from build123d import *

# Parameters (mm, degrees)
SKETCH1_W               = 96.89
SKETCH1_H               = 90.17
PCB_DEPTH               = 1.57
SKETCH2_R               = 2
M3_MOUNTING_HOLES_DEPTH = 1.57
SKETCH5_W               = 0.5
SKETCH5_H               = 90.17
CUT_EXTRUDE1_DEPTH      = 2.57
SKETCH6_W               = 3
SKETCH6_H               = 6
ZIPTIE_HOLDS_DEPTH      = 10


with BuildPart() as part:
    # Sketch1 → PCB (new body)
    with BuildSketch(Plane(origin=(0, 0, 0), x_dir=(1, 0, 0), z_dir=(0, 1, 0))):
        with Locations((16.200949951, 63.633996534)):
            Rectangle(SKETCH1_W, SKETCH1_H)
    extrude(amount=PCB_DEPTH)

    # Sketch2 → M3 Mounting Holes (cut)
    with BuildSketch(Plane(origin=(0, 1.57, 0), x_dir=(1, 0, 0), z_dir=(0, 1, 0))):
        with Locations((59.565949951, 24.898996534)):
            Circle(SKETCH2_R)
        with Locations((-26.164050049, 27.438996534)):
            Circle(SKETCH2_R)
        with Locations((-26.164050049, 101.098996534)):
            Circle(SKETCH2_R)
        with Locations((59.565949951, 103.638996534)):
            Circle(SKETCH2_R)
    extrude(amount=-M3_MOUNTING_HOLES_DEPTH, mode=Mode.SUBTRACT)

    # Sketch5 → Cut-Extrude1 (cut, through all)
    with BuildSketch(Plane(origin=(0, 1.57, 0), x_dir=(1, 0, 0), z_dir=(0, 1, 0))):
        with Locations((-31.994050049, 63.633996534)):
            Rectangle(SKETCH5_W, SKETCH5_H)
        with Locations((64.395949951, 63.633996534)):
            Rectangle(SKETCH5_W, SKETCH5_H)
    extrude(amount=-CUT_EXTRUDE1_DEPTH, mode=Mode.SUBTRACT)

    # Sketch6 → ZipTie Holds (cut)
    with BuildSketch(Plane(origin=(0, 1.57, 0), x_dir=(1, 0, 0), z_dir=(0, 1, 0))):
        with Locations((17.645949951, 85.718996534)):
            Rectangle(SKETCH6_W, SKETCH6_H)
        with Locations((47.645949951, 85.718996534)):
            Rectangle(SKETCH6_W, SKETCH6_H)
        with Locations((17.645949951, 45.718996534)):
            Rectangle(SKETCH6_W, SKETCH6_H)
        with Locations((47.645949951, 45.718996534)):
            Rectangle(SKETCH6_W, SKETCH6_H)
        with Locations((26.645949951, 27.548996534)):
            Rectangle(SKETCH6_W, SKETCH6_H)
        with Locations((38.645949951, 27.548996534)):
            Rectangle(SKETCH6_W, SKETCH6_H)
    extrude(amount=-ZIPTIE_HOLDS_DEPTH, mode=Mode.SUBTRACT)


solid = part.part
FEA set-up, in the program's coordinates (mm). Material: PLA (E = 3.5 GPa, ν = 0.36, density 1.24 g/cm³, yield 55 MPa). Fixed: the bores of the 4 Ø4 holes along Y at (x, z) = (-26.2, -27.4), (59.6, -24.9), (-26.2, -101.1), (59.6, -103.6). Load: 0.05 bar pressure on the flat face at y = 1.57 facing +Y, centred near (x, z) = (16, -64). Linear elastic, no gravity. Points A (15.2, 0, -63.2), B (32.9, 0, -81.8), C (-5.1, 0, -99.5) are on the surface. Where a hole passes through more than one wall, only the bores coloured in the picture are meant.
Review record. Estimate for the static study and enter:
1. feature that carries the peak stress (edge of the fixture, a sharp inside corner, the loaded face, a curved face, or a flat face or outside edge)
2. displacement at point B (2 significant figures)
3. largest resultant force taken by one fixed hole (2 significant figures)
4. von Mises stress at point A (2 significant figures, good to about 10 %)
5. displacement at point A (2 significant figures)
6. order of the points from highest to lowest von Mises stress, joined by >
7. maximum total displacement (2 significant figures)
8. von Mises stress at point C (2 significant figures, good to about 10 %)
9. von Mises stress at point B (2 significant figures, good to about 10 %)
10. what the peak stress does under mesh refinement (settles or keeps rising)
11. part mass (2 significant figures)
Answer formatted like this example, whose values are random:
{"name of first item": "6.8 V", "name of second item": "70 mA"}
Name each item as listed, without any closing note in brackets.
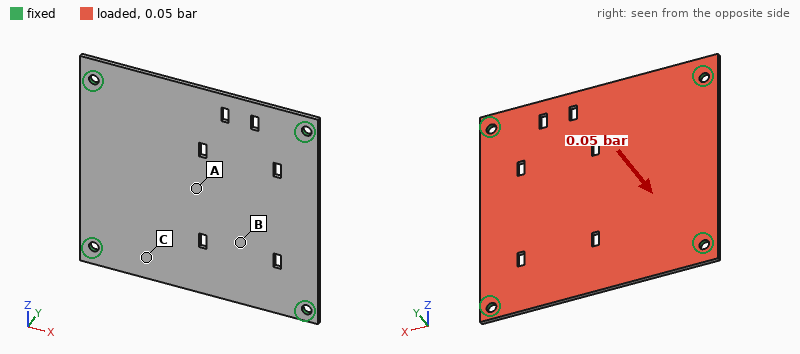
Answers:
{"feature that carries the peak stress": "edge of the fixture", "displacement at point B": "1.0 mm", "largest resultant force taken by one fixed hole": "11 N", "von Mises stress at point A": "4.6 MPa", "displacement at point A": "1.3 mm", "order of the points from highest to lowest von Mises stress, joined by >": "A > B > C", "maximum total displacement": "1.3 mm", "von Mises stress at point C": "1.6 MPa", "von Mises stress at point B": "3.4 MPa", "what the peak stress does under mesh refinement": "keeps rising", "part mass": "17 g"}
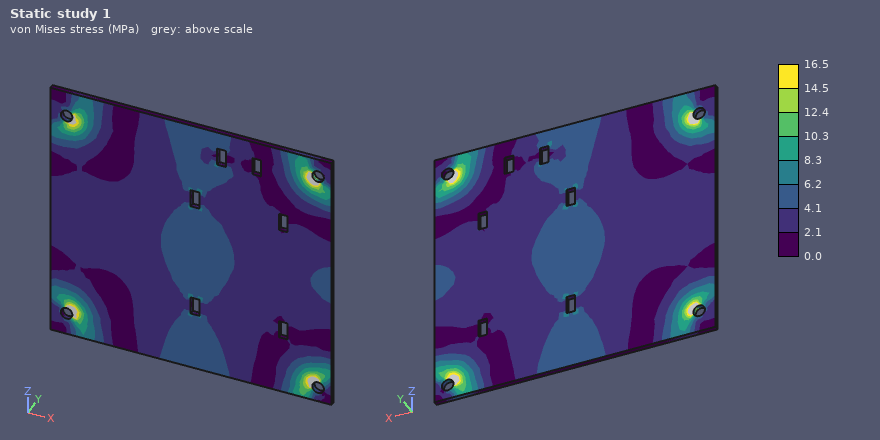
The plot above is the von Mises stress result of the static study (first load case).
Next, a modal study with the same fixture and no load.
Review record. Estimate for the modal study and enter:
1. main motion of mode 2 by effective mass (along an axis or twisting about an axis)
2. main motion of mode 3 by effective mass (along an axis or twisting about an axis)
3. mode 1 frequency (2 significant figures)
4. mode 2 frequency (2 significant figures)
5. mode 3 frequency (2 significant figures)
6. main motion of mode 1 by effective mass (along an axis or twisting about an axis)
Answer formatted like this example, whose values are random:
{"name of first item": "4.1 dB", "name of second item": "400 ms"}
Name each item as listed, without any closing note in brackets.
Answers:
{"main motion of mode 2 by effective mass": "twisting about X", "main motion of mode 3 by effective mass": "twisting about Z", "mode 1 frequency": "270 Hz", "mode 2 frequency": "440 Hz", "mode 3 frequency": "500 Hz", "main motion of mode 1 by effective mass": "along Y"}
